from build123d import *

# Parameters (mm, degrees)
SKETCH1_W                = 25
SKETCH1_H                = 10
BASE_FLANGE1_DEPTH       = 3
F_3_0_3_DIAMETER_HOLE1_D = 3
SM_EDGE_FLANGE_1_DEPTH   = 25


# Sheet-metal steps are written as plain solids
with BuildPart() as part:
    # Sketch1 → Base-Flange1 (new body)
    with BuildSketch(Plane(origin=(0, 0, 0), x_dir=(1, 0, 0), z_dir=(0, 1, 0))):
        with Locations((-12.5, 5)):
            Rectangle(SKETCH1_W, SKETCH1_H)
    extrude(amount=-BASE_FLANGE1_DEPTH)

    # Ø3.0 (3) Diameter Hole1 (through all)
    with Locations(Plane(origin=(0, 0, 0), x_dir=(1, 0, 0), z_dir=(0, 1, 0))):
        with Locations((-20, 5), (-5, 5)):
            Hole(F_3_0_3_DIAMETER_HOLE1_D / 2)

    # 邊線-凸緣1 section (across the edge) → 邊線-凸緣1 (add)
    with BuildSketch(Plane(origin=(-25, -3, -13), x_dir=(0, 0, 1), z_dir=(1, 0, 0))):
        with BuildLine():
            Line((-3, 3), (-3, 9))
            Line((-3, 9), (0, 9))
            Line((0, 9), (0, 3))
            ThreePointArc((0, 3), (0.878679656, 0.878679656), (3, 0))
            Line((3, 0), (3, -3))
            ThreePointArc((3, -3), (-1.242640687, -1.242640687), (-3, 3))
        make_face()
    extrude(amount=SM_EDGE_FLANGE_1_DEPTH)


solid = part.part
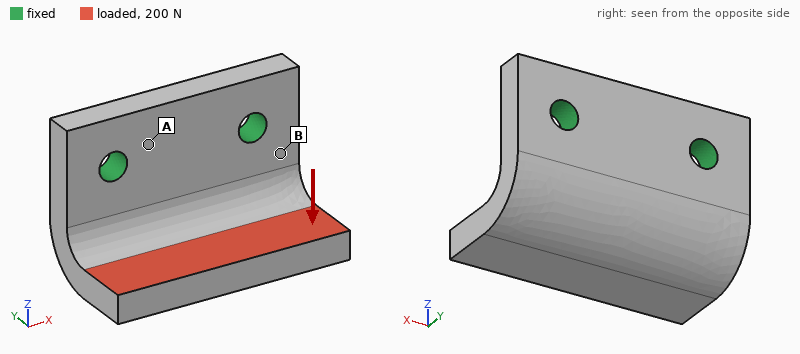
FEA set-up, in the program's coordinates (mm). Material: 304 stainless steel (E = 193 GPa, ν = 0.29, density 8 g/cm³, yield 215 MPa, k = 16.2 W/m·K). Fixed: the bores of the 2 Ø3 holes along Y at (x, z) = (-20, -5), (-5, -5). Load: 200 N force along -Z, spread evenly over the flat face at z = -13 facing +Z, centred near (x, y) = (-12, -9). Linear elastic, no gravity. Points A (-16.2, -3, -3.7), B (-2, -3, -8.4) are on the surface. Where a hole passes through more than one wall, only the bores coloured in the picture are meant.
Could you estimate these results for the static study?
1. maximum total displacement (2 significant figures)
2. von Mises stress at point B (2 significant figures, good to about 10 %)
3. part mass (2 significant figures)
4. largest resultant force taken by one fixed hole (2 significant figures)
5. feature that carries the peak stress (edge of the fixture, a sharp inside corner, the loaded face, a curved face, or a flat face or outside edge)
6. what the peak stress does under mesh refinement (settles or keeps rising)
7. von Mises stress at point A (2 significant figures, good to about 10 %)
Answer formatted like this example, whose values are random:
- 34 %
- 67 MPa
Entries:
- 16 µm
- 39 MPa
- 14 g
- 100 N
- edge of the fixture
- keeps rising
- 11 MPa
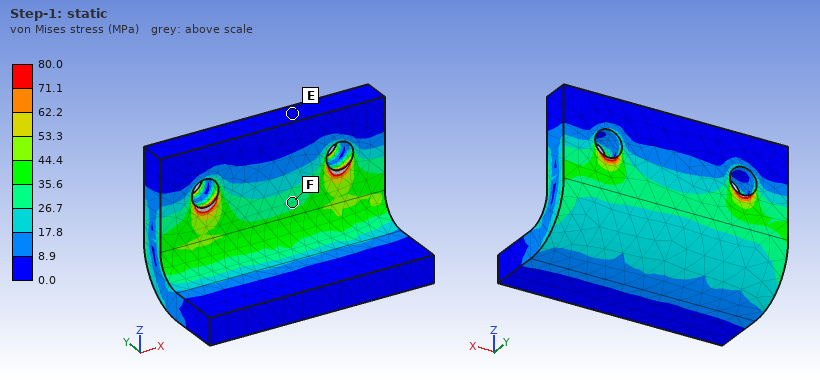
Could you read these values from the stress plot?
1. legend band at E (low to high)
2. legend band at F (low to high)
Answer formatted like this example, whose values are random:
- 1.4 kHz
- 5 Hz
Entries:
- 0.0 to 8.9 MPa
- 26.7 to 35.6 MPa
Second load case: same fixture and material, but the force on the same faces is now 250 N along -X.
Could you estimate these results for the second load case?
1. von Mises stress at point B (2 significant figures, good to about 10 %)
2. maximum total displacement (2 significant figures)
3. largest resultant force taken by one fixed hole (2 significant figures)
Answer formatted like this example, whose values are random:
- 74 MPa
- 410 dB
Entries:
- 21 MPa
- 7.4 µm
- 200 N
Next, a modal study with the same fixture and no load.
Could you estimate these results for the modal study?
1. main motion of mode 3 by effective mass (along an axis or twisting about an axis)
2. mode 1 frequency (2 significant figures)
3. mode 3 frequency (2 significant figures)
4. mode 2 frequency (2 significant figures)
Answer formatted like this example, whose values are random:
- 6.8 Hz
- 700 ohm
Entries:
- along Y
- 8600 Hz
- 26 kHz
- 14 kHz
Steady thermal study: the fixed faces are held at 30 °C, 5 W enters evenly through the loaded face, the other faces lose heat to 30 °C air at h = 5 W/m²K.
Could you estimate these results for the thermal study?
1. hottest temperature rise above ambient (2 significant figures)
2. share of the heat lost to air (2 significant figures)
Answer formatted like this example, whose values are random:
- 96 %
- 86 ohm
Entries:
- 63 K
- 3.4 %
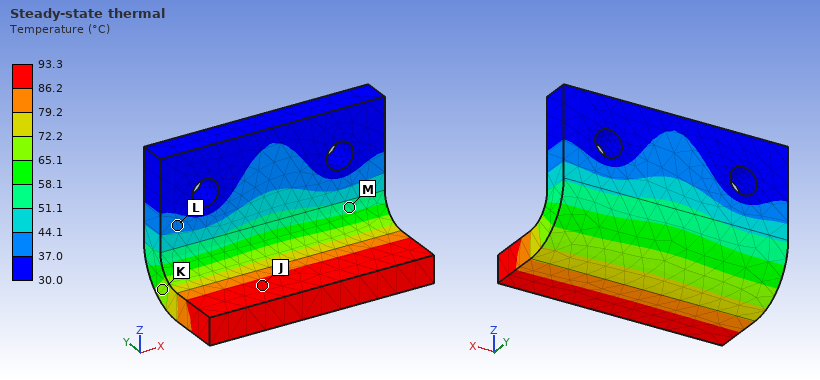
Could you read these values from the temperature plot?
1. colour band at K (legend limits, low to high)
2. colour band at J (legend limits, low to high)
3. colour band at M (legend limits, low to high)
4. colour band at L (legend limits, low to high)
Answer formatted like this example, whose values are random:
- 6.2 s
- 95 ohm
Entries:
- 65.1 to 72.2 °C
- 86.2 to 93.3 °C
- 51.1 to 58.1 °C
- 37.0 to 44.1 °C
